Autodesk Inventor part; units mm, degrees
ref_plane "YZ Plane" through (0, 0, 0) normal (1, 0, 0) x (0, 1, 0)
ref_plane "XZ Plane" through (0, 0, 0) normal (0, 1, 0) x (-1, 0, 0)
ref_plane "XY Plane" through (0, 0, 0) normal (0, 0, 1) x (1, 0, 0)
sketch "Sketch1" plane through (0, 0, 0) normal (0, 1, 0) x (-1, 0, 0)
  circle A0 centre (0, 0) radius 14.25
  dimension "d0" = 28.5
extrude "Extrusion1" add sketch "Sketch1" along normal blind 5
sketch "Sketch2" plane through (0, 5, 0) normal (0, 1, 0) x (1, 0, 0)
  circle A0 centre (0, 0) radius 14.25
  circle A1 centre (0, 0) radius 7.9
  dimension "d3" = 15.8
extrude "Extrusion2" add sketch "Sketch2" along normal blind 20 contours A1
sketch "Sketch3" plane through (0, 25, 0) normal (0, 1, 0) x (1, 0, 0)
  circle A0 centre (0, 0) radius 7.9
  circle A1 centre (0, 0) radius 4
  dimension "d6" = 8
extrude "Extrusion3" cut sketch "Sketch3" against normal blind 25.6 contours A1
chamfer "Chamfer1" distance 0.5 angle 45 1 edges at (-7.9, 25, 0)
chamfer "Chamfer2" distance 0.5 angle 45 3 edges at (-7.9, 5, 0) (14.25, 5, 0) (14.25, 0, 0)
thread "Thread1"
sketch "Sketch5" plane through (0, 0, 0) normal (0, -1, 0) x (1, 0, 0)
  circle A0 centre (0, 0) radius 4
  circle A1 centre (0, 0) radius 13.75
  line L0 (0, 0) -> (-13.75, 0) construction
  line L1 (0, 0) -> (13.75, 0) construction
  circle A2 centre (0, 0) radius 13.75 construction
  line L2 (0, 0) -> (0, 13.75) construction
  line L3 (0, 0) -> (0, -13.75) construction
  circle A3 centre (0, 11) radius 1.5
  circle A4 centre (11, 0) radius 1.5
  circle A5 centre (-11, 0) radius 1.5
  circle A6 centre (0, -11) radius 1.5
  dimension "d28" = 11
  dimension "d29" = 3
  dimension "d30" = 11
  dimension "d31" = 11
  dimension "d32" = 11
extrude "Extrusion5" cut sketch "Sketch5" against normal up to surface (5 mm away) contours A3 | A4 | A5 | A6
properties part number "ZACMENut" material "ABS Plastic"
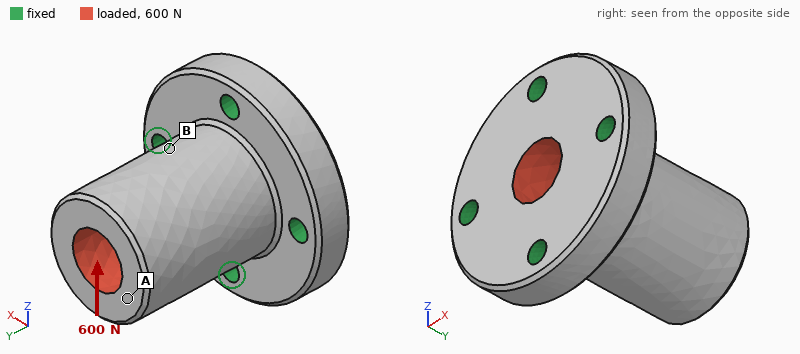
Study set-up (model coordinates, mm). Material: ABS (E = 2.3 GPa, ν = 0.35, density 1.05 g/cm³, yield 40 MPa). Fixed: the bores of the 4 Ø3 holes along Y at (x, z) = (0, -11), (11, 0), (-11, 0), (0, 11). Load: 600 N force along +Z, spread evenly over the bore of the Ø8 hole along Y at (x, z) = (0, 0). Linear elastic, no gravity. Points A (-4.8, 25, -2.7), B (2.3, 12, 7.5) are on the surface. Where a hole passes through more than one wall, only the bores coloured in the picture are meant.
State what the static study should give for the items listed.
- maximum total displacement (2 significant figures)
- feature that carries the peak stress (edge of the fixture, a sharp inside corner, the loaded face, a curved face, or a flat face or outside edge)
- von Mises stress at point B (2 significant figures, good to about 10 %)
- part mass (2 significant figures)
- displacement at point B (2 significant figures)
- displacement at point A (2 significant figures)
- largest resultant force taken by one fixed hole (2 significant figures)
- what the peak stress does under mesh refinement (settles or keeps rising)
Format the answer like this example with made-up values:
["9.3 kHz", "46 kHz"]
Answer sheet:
["0.24 mm", "a sharp inside corner", "5.1 MPa", "6.0 g", "0.11 mm", "0.23 mm", "350 N", "keeps rising"]
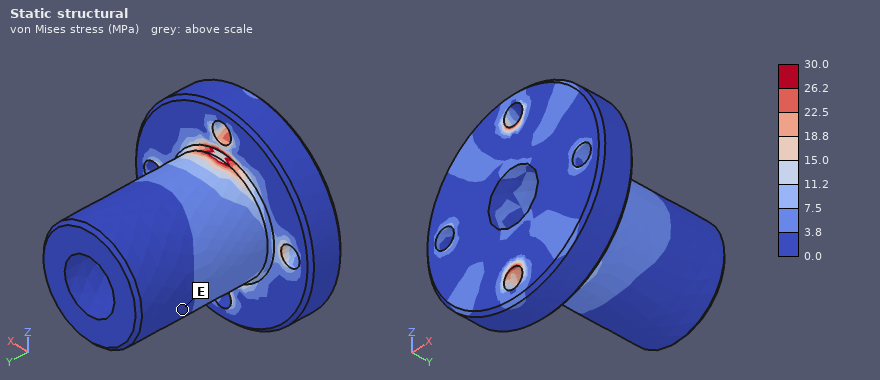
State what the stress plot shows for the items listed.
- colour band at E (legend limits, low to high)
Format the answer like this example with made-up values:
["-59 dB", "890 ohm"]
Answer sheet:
["0.0 to 3.8 MPa"]
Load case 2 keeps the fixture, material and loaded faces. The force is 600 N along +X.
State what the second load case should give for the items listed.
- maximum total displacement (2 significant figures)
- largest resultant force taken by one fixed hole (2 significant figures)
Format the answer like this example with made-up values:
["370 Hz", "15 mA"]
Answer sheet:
["0.24 mm", "350 N"]
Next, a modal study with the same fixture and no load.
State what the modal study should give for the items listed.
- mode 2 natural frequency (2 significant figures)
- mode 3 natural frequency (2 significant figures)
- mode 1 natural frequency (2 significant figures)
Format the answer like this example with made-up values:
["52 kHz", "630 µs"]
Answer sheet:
["4900 Hz", "10 kHz", "4900 Hz"]
